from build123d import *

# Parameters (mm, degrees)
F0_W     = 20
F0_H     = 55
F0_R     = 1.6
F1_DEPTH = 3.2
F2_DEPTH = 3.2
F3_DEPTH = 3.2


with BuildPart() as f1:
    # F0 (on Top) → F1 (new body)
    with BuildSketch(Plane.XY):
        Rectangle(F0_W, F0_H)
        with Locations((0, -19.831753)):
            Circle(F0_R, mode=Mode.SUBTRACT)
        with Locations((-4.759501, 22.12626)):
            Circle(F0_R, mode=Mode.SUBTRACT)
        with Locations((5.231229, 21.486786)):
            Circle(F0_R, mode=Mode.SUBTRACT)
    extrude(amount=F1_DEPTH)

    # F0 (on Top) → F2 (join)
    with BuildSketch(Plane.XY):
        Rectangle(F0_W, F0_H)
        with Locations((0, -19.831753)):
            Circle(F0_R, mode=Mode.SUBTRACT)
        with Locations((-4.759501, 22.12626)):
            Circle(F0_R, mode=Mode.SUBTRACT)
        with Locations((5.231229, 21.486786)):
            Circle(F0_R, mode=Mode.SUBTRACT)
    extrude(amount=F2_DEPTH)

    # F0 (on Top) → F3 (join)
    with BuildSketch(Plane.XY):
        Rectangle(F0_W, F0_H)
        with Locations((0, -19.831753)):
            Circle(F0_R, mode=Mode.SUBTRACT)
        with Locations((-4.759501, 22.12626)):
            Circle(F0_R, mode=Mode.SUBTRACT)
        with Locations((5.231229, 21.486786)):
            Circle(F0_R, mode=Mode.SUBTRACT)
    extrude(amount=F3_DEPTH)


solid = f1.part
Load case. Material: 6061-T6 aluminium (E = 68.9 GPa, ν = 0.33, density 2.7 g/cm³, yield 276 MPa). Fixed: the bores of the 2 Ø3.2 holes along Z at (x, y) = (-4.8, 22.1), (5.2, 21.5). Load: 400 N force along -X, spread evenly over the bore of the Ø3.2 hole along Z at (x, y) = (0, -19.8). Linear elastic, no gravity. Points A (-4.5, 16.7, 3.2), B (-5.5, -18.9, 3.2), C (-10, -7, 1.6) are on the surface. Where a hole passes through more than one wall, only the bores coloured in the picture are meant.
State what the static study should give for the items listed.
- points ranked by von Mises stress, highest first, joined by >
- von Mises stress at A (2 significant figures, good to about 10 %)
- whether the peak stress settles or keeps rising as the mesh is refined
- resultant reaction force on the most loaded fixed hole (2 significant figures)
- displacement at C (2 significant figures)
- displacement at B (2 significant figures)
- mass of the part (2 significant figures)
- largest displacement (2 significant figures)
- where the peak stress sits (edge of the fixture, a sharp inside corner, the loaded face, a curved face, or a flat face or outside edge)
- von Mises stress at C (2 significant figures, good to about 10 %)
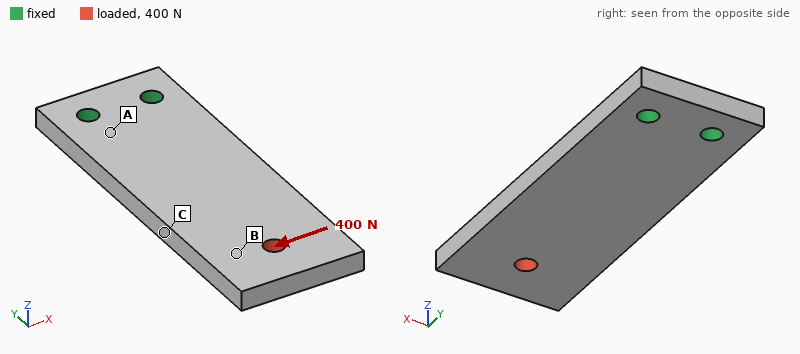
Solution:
A > C > B
46 MPa
keeps rising
1.4 kN
0.055 mm
0.083 mm
9.3 g
0.11 mm
edge of the fixture
24 MPa
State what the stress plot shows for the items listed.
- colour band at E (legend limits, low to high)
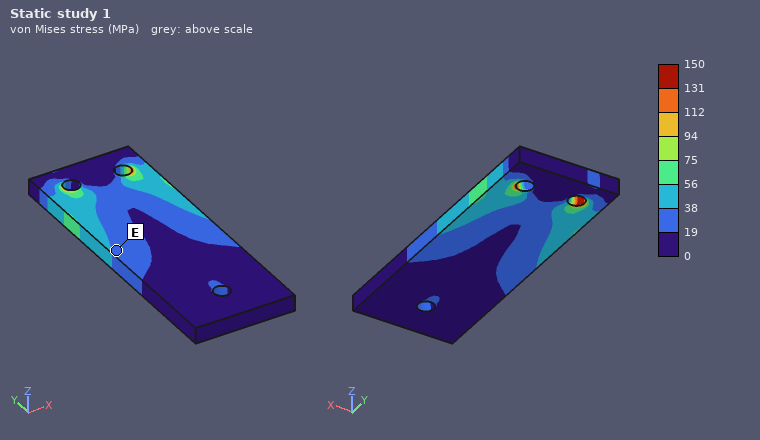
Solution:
19 to 38 MPa
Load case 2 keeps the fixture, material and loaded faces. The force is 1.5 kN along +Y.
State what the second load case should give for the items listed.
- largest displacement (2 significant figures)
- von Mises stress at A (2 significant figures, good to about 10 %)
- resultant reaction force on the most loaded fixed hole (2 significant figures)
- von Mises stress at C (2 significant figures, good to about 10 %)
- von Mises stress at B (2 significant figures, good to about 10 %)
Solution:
18 µm
28 MPa
780 N
22 MPa
17 MPa
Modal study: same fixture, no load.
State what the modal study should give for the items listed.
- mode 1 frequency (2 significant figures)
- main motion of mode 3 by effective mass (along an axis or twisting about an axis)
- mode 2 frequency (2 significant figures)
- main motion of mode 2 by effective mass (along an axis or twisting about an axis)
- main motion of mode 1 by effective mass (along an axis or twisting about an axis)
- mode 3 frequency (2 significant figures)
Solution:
1100 Hz
along X
5200 Hz
twisting about Y
along Z
5700 Hz
